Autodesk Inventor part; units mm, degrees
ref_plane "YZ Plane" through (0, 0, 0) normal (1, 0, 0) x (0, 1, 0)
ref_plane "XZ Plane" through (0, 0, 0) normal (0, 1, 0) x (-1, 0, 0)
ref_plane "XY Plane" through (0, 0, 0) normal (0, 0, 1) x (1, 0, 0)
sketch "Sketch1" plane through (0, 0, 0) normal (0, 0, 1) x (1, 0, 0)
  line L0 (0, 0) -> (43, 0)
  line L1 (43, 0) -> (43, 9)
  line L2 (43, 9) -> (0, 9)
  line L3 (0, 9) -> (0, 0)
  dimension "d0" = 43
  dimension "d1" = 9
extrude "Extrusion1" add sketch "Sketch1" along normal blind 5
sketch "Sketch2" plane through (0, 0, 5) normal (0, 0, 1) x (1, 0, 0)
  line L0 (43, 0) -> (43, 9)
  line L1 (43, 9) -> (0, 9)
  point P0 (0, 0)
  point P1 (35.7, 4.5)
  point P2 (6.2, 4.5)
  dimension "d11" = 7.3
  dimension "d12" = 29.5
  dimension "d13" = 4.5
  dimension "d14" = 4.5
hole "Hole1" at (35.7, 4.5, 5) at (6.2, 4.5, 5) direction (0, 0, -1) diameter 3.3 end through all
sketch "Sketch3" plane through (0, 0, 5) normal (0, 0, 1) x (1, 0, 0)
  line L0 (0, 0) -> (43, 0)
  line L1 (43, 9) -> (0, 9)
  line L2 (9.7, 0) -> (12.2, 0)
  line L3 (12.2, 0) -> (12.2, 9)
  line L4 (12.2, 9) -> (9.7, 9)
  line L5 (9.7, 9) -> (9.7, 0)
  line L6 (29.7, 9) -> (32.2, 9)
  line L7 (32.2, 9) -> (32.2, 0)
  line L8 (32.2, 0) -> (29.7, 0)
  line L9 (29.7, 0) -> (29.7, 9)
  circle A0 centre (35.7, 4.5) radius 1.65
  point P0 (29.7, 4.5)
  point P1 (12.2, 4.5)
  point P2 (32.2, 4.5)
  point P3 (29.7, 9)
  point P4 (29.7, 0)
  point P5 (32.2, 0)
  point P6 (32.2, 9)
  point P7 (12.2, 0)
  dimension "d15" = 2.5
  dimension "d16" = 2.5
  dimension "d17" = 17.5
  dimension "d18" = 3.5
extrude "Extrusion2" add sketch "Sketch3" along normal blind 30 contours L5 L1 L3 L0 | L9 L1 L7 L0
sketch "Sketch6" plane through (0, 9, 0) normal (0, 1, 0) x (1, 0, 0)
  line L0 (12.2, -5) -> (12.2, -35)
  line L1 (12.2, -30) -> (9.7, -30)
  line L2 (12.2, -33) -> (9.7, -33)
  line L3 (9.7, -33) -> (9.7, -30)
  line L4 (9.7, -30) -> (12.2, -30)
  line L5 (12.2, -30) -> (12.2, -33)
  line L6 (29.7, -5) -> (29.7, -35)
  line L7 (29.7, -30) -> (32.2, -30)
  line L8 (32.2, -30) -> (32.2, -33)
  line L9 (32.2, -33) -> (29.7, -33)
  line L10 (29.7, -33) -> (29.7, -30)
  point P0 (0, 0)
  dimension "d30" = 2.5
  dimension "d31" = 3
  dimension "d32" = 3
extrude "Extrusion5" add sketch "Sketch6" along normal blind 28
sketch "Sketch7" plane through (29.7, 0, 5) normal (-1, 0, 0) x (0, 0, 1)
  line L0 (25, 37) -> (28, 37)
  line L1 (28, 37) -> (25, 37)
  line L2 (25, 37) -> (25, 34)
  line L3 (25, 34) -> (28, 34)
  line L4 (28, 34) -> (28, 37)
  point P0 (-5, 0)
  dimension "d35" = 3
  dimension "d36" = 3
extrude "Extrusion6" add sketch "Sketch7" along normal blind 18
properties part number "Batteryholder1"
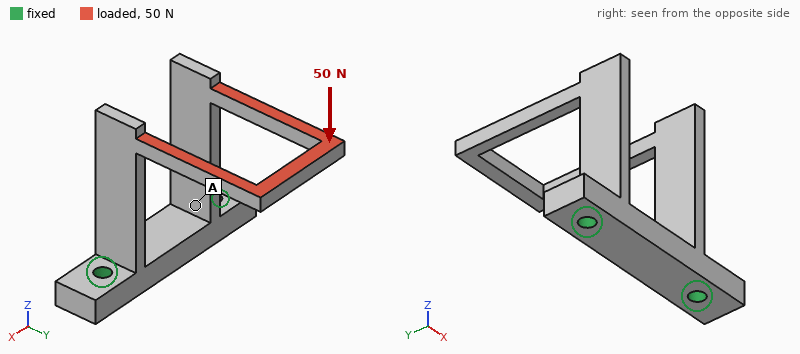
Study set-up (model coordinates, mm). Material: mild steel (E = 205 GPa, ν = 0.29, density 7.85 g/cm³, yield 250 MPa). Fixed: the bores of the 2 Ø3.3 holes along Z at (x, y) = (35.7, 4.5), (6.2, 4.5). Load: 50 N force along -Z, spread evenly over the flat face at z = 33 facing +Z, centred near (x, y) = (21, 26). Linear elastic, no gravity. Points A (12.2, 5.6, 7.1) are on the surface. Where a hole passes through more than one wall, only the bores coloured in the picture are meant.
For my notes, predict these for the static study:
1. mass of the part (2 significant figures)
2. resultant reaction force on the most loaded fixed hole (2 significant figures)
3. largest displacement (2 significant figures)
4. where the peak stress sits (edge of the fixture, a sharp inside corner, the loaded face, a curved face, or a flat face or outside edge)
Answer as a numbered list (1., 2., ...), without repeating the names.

1. 30 g
2. 25 N
3. 0.12 mm
4. the loaded face
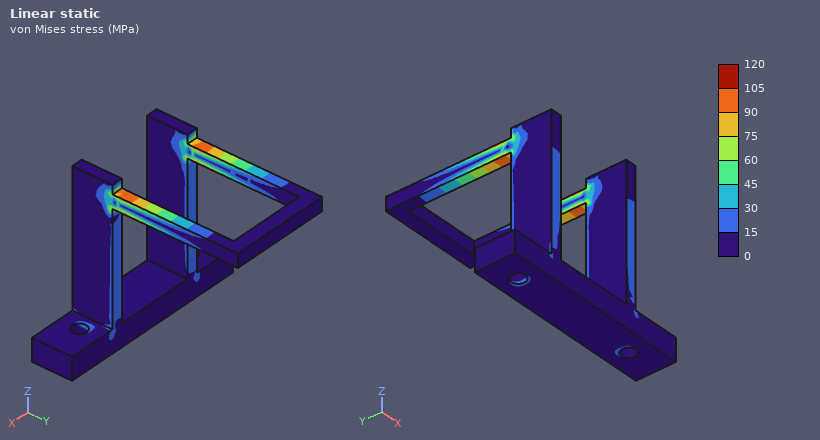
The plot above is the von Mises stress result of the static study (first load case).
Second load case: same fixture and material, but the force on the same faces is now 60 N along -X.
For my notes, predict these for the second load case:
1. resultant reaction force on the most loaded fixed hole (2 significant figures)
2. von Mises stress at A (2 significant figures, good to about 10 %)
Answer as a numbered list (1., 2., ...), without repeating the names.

1. 75 N
2. 80 MPa
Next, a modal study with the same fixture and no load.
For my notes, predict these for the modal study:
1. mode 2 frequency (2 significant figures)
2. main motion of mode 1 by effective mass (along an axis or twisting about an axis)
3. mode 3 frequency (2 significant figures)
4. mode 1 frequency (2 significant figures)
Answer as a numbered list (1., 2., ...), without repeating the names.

1. 1700 Hz
2. along X
3. 2400 Hz
4. 1300 Hz
